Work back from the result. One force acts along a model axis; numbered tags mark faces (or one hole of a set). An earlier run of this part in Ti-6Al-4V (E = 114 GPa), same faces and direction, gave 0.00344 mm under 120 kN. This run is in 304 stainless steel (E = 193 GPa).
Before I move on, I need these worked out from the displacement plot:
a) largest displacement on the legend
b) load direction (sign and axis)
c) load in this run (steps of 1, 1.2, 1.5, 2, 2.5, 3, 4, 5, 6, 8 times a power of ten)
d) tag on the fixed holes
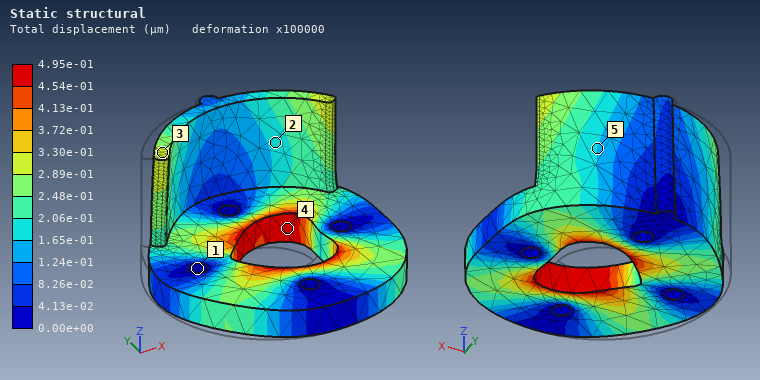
4.95e-01 µm
+X
30 kN
1
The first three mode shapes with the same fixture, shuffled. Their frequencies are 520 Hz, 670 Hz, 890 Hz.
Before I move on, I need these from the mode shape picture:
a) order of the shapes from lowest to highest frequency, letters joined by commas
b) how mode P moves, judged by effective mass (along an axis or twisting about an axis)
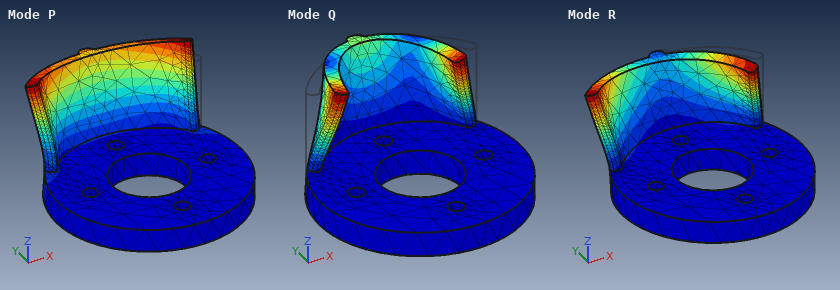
R, P, Q
along Y
